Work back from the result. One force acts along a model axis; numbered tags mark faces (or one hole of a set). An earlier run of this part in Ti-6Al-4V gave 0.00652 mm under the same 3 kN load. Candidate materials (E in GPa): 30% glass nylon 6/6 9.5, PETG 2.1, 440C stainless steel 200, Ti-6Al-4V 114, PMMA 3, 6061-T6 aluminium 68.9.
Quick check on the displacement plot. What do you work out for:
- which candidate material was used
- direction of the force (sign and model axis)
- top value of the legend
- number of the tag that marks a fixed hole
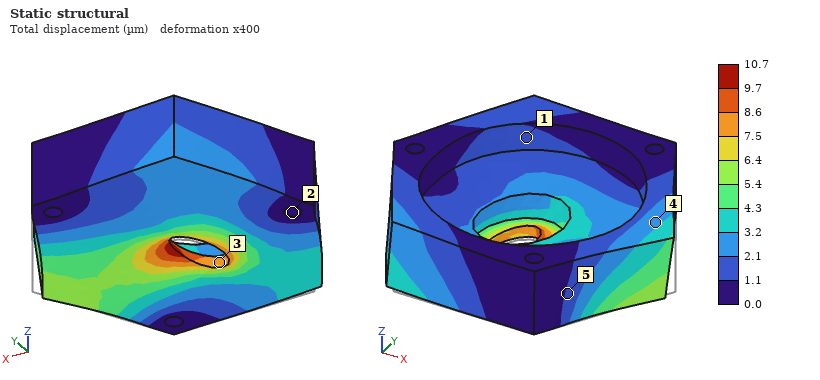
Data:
6061-T6 aluminium
-X
10.7 µm
2
